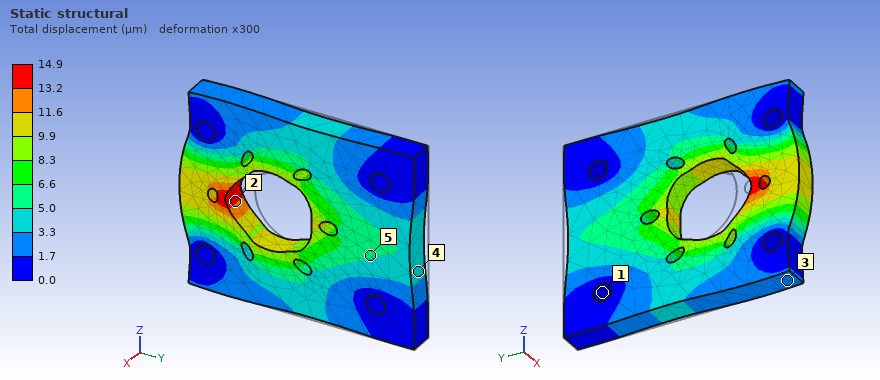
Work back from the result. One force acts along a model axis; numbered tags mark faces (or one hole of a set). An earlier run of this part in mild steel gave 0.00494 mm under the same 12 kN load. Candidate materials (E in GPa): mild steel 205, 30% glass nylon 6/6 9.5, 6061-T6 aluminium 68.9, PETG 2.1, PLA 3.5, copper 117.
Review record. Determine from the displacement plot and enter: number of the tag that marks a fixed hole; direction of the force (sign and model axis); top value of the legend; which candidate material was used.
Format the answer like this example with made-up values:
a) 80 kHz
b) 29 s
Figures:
a) 1
b) -Y
c) 14.9 µm
d) 6061-T6 aluminium
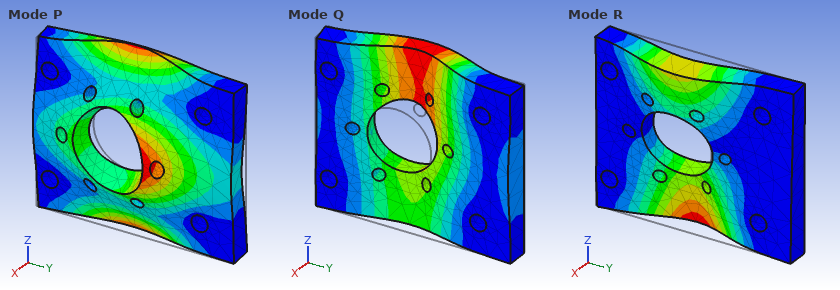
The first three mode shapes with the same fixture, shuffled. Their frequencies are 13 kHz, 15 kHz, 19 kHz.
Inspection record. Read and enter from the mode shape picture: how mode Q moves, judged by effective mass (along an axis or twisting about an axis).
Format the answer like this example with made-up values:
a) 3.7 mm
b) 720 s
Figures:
a) along X
